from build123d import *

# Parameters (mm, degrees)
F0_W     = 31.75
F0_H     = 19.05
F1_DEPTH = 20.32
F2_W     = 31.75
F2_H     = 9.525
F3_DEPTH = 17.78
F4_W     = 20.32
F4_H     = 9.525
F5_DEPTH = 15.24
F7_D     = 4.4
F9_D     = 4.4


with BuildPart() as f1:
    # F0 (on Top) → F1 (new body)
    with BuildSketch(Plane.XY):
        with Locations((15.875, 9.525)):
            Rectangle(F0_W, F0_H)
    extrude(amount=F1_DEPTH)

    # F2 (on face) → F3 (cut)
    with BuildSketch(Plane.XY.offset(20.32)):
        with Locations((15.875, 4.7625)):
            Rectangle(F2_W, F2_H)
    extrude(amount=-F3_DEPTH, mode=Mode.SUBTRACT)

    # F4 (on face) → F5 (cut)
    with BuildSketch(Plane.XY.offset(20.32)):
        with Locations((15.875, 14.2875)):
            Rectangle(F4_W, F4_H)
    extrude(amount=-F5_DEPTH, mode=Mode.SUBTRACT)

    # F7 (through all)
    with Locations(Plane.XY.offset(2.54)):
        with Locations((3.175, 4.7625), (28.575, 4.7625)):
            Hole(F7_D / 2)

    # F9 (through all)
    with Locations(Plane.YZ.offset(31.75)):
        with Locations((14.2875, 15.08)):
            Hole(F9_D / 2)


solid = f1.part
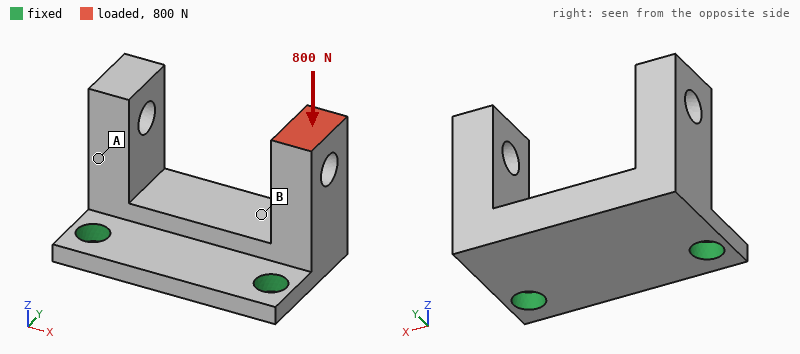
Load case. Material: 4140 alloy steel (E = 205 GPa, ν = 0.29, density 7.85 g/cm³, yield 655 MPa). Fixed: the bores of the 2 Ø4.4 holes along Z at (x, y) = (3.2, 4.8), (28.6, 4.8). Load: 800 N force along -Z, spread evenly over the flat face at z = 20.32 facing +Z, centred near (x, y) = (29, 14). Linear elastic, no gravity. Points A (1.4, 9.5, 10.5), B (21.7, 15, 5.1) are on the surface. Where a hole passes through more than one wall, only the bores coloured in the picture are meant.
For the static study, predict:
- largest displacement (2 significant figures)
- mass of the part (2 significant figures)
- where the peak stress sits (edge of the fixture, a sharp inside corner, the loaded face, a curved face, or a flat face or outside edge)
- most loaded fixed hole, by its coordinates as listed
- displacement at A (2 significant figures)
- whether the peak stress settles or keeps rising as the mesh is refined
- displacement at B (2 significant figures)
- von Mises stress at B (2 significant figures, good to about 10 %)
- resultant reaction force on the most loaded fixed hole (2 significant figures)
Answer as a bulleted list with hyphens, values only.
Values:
- 92 µm
- 29 g
- edge of the fixture
- (28.6, 4.8)
- 22 µm
- keeps rising
- 30 µm
- 61 MPa
- 800 N
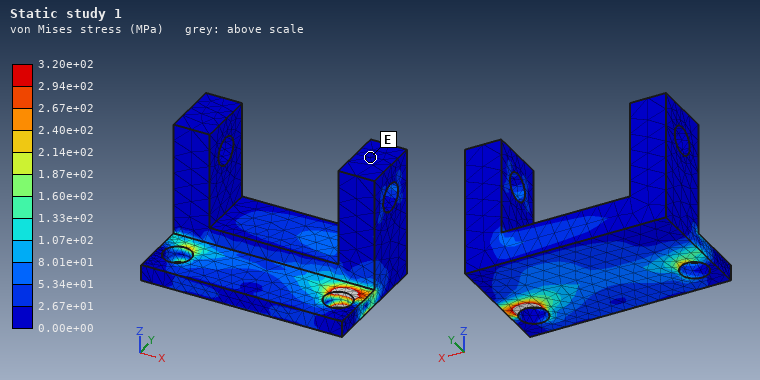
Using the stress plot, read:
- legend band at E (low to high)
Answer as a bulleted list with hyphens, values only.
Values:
- 0.00e+00 to 2.67e+01 MPa
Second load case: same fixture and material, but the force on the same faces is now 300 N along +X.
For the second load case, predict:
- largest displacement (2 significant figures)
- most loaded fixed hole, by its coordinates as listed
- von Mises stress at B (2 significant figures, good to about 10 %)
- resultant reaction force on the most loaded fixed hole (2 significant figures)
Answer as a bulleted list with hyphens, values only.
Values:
- 48 µm
- (3.2, 4.8)
- 68 MPa
- 320 N
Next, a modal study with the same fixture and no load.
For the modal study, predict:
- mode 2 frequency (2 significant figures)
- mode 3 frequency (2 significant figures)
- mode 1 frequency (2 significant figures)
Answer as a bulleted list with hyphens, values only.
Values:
- 6600 Hz
- 8600 Hz
- 3600 Hz
